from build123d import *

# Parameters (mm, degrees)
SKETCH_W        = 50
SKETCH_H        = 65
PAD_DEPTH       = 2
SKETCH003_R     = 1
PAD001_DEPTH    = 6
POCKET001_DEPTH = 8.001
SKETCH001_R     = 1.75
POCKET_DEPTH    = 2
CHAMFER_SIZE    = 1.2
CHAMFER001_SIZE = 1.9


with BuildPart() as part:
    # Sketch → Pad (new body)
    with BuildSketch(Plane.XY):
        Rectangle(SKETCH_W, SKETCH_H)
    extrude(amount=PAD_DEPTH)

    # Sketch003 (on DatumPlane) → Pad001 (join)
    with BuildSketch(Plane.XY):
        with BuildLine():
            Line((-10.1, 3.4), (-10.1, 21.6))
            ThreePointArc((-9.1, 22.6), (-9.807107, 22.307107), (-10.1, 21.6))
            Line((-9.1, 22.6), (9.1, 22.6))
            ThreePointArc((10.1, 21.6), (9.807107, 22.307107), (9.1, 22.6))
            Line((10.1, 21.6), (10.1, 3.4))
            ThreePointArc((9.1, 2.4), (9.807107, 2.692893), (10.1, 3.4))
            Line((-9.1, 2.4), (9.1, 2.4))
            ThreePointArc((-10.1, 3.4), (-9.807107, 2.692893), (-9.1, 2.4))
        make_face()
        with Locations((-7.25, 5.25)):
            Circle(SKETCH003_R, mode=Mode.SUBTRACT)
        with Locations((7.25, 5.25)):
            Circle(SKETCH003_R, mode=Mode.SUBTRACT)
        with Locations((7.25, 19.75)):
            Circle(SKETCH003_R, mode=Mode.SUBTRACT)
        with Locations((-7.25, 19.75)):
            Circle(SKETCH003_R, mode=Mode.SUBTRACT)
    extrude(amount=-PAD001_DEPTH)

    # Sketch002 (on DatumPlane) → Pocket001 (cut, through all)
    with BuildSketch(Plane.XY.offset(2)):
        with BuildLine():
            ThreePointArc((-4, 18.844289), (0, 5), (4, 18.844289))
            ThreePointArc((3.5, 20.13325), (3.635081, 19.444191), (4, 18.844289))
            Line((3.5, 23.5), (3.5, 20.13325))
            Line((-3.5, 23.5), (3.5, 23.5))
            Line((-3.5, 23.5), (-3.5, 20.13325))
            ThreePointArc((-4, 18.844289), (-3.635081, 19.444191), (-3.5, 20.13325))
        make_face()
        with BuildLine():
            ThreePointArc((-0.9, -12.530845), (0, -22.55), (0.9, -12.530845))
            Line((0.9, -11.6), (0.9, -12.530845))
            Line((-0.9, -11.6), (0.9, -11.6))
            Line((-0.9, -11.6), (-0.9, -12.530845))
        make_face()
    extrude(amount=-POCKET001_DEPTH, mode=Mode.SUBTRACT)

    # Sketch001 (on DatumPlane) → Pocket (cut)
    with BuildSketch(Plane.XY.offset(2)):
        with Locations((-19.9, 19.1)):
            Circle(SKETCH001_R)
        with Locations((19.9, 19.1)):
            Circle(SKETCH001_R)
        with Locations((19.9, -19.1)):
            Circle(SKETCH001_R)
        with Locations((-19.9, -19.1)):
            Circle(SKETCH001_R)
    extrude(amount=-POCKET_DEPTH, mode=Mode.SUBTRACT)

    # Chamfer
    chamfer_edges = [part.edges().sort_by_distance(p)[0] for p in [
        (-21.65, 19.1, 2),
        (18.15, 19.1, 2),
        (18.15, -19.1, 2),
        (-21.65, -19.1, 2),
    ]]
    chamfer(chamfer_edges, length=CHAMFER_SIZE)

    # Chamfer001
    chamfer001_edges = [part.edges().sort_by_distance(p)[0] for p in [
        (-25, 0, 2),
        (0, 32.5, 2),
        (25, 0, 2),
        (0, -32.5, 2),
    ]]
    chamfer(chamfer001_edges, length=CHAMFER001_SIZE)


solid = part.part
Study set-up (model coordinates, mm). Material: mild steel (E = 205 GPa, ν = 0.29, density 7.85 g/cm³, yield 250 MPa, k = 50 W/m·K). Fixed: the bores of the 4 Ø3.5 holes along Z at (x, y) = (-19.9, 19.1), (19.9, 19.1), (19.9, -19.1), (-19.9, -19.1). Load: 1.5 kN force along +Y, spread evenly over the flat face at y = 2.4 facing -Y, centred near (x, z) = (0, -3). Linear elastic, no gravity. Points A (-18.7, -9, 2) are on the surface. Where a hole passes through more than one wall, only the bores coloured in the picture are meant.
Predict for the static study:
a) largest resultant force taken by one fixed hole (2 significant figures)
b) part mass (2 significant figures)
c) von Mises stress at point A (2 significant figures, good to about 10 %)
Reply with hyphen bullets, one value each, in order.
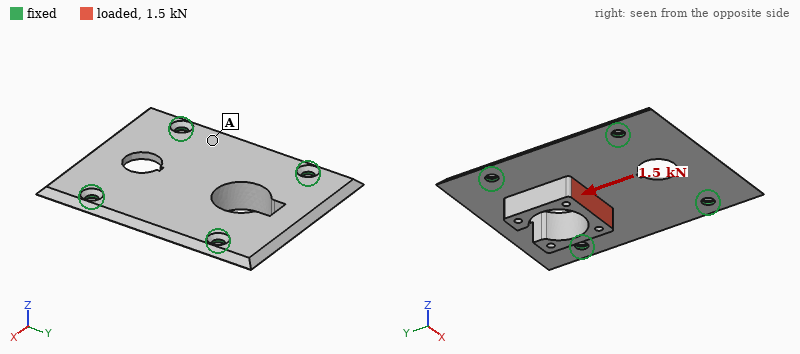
- 550 N
- 52 g
- 19 MPa
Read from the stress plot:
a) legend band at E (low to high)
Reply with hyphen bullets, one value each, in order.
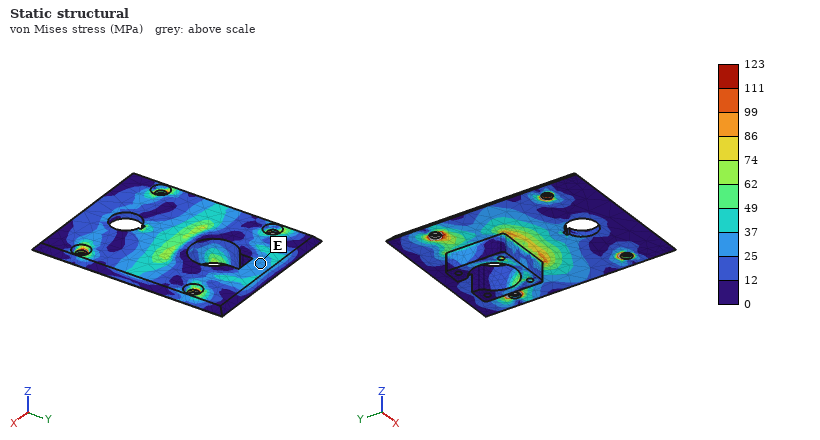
- 25 to 37 MPa
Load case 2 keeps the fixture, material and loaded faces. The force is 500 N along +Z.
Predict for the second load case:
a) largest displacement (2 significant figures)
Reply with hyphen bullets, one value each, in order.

- 52 µm
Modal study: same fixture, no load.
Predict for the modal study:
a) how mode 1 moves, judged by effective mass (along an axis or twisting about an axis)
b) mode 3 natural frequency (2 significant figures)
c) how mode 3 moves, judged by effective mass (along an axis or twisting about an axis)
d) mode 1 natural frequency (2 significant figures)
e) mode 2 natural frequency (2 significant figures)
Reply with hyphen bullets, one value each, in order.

- along Z
- 5200 Hz
- along Z
- 4200 Hz
- 5000 Hz
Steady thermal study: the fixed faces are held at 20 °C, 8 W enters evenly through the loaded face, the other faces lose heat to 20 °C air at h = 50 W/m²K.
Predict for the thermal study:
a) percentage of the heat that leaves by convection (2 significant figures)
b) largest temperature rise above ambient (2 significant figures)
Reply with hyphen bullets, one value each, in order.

- 36 %
- 31 K
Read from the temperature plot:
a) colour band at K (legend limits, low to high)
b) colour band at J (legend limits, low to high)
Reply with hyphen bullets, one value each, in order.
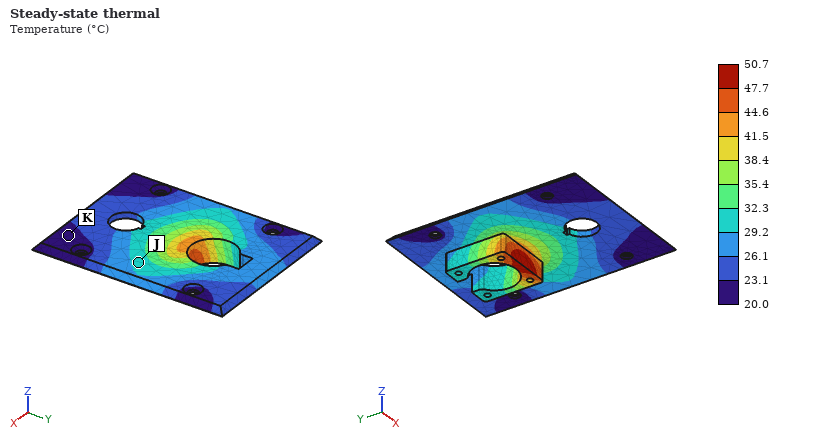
- 20.0 to 23.1 °C
- 29.2 to 32.3 °C
